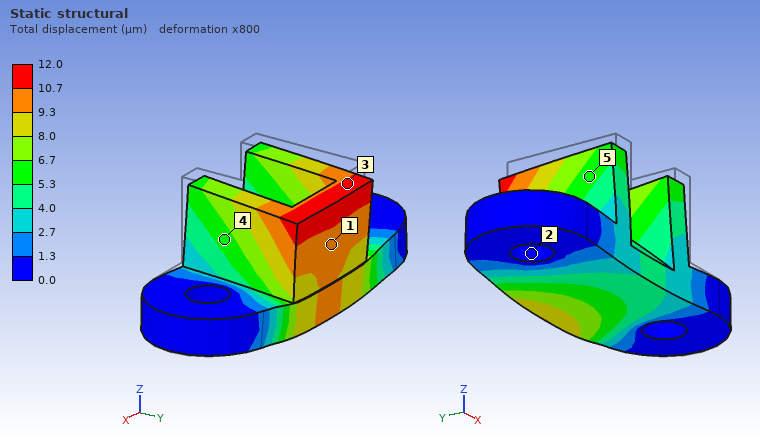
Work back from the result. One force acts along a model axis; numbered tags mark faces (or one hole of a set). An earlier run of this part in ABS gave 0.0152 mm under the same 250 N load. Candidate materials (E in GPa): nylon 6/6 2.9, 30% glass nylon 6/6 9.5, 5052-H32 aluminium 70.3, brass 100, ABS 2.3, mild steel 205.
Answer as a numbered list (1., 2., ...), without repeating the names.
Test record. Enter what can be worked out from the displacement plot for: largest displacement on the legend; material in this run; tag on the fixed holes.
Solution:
1. 12.0 µm
2. nylon 6/6
3. 2
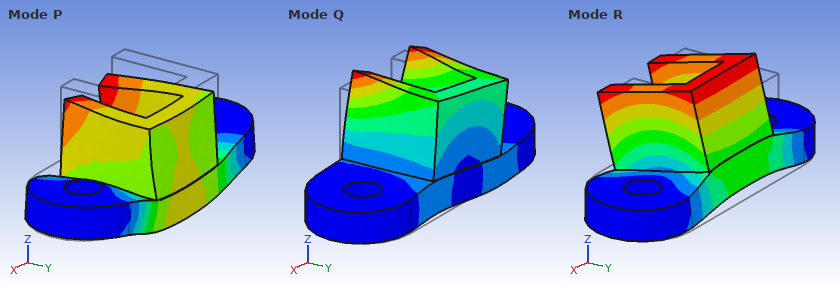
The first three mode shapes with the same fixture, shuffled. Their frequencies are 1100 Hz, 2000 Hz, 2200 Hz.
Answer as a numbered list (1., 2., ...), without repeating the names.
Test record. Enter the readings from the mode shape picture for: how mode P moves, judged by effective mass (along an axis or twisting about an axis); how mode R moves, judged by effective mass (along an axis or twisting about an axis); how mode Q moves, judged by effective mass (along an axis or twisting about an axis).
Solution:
1. along Z
2. along Y
3. along X
